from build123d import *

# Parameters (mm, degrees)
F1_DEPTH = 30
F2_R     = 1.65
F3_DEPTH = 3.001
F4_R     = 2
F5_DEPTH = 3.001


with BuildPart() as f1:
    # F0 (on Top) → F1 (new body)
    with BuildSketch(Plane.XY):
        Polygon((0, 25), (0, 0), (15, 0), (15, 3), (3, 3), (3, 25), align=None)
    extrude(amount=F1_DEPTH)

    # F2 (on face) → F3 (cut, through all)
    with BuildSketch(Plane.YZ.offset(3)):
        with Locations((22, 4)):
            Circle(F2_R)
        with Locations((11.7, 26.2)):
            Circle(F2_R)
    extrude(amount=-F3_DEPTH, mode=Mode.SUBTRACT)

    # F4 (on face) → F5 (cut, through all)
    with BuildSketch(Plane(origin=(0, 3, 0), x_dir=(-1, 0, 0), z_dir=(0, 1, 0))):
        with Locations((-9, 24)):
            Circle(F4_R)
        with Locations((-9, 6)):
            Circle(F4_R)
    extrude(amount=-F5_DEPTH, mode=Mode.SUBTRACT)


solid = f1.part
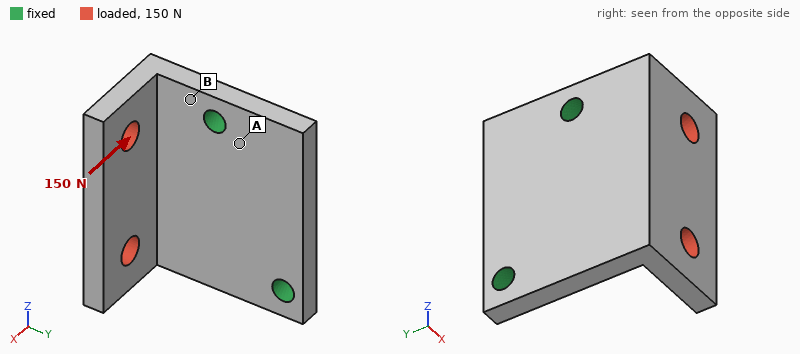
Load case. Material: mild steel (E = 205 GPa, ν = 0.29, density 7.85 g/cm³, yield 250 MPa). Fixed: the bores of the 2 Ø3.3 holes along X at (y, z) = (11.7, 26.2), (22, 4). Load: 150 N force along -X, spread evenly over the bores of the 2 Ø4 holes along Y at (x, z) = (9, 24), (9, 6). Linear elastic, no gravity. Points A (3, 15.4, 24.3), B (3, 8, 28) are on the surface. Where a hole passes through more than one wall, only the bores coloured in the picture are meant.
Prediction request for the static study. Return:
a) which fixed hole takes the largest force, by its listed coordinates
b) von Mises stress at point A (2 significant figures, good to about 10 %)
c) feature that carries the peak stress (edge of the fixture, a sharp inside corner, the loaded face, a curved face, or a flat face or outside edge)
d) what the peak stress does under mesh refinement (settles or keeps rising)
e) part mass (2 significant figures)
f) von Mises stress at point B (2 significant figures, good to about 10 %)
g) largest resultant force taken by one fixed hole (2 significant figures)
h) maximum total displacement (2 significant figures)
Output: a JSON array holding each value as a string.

["(11.7, 26.2)", "12 MPa", "edge of the fixture", "keeps rising", "25 g", "41 MPa", "110 N", "26 µm"]
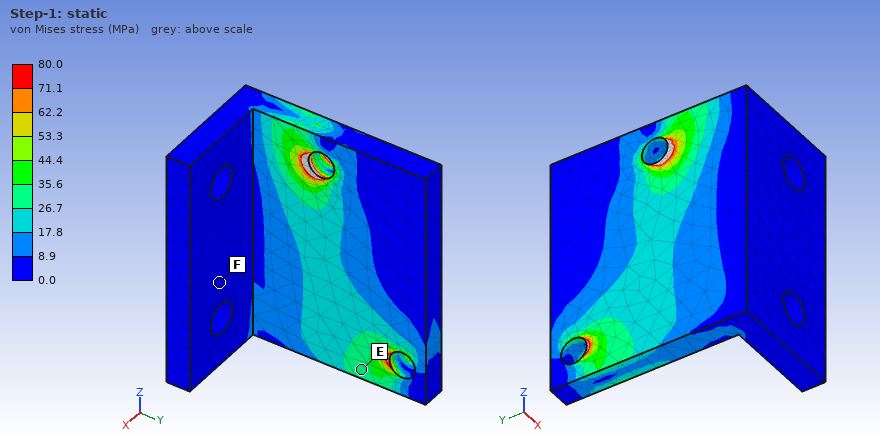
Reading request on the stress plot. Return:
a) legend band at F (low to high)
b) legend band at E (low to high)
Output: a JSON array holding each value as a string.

["0.0 to 8.9 MPa", "26.7 to 35.6 MPa"]
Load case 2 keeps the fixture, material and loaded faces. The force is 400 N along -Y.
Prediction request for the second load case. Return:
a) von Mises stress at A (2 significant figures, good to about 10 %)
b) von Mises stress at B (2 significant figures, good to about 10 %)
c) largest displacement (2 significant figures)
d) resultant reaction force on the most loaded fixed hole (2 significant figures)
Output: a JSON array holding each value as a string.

["17 MPa", "95 MPa", "58 µm", "210 N"]
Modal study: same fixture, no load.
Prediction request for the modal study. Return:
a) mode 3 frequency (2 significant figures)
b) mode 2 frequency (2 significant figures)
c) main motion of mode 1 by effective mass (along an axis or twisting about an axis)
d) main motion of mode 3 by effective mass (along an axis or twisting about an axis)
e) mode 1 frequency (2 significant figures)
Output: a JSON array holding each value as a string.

["13 kHz", "7900 Hz", "along X", "along X", "4000 Hz"]
